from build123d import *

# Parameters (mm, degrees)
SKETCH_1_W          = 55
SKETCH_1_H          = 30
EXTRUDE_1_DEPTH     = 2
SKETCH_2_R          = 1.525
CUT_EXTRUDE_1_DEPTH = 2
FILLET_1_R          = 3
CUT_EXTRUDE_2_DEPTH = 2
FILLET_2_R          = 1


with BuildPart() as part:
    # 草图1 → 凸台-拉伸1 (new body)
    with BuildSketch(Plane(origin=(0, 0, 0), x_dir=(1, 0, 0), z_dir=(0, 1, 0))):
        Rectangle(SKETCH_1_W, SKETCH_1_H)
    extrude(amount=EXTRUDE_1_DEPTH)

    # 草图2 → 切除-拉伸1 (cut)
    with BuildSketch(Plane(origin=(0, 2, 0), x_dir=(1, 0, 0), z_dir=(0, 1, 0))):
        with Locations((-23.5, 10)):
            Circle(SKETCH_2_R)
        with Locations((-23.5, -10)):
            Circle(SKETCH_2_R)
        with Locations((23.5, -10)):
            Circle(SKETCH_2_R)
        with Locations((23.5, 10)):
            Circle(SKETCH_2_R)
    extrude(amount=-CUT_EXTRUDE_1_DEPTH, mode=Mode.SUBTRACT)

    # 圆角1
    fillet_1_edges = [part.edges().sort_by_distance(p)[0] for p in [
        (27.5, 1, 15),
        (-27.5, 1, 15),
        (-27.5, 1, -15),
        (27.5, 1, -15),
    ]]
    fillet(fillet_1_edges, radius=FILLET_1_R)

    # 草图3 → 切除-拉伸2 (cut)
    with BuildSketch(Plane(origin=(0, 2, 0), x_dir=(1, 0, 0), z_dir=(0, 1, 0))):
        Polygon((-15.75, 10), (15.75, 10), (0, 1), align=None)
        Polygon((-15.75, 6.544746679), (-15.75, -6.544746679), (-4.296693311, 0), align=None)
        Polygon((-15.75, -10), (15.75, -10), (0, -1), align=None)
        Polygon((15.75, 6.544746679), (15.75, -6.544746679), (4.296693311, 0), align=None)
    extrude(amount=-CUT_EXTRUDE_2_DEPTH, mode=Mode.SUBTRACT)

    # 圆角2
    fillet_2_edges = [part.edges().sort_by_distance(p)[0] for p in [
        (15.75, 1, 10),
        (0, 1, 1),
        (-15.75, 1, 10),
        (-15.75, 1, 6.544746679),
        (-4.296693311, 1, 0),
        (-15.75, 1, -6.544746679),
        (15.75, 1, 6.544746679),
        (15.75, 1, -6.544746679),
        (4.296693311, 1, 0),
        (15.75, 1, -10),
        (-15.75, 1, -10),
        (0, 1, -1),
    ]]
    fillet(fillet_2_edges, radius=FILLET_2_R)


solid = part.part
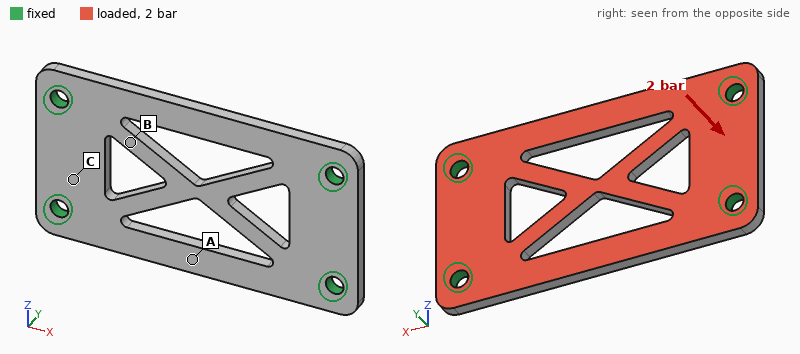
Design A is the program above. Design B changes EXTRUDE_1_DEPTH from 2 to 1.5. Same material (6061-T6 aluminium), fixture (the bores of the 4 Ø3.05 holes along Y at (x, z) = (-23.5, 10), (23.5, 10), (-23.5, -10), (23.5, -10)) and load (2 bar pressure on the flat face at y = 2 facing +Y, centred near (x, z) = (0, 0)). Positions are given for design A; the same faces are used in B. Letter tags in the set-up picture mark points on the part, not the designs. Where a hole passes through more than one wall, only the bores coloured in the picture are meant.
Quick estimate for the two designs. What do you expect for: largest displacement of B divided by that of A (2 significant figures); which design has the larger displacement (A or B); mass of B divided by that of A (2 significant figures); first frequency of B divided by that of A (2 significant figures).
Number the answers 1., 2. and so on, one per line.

1. 2.3
2. B
3. 0.75
4. 0.77
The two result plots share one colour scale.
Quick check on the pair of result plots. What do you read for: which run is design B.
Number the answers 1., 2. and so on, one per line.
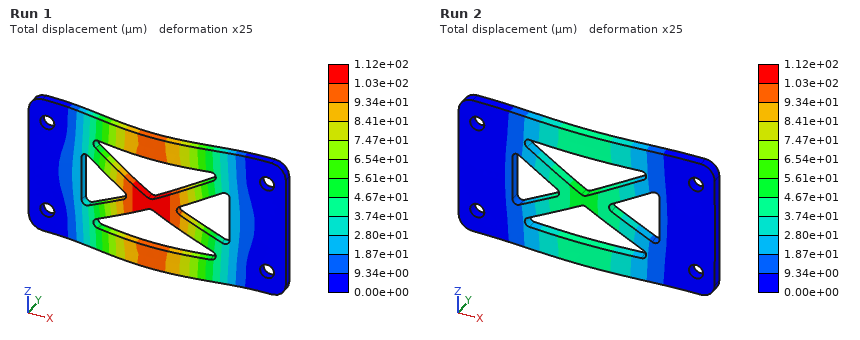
1. Run 1
